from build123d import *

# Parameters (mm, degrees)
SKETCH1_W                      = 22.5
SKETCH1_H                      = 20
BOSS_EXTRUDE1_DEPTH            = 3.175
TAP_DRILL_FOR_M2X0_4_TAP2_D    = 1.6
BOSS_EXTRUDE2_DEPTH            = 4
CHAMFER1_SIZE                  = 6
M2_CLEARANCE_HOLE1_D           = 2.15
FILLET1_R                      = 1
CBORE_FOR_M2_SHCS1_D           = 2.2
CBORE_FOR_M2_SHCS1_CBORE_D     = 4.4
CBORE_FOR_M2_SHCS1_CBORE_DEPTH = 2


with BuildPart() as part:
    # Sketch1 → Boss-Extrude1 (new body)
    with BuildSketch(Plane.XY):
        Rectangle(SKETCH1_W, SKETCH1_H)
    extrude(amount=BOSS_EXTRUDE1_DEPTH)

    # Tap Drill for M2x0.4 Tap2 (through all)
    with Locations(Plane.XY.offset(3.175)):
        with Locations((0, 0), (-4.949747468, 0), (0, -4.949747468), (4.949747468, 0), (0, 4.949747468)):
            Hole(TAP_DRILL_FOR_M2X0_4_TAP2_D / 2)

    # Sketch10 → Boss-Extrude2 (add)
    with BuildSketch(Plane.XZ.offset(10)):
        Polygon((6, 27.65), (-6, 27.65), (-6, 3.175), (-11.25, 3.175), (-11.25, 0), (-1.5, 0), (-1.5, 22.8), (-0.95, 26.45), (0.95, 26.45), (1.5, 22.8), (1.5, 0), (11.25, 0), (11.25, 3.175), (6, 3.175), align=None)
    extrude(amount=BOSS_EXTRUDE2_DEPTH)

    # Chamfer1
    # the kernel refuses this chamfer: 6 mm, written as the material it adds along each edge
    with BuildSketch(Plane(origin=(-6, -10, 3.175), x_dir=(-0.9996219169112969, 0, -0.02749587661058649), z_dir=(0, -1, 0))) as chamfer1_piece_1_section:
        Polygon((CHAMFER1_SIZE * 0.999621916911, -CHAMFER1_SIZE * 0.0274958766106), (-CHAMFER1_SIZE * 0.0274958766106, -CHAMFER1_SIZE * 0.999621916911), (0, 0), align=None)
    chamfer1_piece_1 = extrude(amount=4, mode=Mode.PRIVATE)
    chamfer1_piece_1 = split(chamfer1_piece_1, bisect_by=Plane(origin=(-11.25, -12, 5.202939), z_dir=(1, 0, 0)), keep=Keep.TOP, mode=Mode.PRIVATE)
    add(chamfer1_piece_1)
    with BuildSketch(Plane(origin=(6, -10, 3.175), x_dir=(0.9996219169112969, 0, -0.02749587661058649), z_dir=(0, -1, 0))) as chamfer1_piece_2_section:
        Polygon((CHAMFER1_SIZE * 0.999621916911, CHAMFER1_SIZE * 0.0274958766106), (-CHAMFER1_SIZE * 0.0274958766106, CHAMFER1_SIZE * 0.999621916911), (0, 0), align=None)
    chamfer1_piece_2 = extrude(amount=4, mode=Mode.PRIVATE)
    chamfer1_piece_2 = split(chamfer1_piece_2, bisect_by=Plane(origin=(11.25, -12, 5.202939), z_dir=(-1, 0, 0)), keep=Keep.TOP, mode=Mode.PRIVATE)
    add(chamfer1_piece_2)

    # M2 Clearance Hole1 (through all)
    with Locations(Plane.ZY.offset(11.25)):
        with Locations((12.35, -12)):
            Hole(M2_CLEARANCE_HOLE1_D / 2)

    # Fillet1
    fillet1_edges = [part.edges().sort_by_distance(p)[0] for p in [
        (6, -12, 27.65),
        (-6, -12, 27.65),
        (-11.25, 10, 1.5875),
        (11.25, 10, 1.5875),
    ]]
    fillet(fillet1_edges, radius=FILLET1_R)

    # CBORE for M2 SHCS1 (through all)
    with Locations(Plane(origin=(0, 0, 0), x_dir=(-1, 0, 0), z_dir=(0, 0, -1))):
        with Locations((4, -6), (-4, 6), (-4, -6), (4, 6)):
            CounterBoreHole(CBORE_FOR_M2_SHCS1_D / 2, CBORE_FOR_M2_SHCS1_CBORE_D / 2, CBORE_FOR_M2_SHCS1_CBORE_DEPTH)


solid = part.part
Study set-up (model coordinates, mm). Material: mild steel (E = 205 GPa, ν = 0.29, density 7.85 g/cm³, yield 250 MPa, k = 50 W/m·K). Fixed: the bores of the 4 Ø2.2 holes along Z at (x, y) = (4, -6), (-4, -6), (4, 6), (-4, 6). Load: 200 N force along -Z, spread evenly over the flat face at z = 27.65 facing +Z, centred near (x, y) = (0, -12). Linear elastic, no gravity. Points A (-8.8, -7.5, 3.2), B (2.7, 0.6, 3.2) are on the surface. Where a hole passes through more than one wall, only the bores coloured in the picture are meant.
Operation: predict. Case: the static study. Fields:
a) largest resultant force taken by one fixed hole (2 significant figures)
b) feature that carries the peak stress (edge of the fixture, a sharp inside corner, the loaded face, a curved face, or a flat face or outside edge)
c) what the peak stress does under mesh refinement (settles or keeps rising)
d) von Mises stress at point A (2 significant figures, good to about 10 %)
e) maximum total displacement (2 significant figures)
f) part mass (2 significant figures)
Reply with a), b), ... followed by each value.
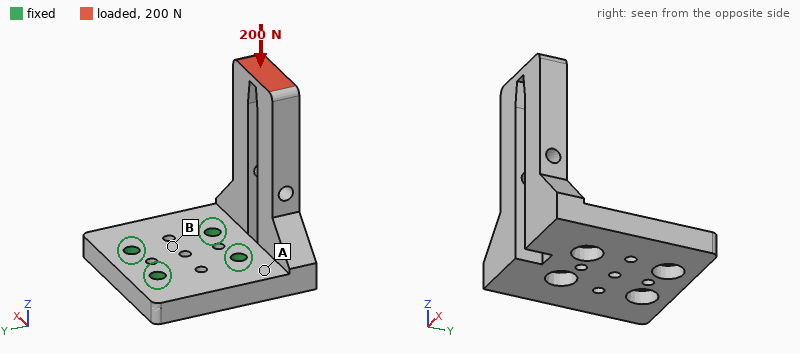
a) 150 N
b) edge of the fixture
c) keeps rising
d) 20 MPa
e) 18 µm
f) 20 g
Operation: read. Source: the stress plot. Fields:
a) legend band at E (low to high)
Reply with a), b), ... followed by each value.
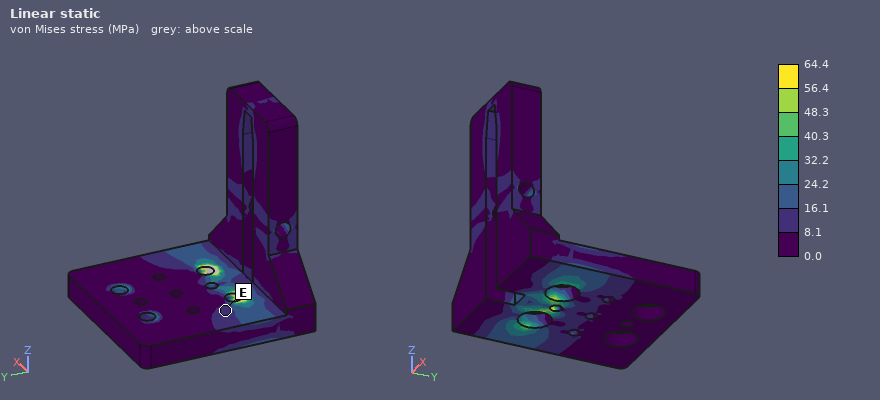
a) 8.1 to 16.1 MPa
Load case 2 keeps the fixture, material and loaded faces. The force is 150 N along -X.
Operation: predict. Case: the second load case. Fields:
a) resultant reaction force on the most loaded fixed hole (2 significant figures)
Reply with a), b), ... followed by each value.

a) 410 N
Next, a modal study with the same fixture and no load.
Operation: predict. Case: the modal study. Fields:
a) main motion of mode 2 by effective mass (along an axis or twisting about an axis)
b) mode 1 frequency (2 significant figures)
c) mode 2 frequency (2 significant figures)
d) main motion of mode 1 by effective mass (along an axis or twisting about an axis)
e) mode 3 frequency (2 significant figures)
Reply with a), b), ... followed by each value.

a) along X
b) 3400 Hz
c) 5700 Hz
d) along Y
e) 13 kHz
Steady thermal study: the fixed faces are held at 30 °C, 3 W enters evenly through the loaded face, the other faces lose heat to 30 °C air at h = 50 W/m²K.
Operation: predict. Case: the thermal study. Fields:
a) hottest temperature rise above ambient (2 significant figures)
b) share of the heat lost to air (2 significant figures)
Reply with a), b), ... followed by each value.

a) 41 K
b) 36 %
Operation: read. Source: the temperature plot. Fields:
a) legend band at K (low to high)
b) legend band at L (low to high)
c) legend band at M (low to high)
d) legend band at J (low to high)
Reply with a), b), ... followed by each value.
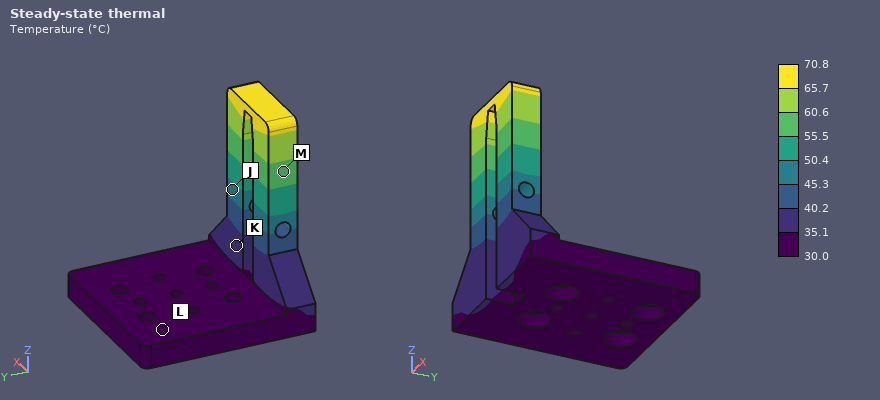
a) 35.1 to 40.2 °C
b) 30.0 to 35.1 °C
c) 55.5 to 60.6 °C
d) 45.3 to 50.4 °C
